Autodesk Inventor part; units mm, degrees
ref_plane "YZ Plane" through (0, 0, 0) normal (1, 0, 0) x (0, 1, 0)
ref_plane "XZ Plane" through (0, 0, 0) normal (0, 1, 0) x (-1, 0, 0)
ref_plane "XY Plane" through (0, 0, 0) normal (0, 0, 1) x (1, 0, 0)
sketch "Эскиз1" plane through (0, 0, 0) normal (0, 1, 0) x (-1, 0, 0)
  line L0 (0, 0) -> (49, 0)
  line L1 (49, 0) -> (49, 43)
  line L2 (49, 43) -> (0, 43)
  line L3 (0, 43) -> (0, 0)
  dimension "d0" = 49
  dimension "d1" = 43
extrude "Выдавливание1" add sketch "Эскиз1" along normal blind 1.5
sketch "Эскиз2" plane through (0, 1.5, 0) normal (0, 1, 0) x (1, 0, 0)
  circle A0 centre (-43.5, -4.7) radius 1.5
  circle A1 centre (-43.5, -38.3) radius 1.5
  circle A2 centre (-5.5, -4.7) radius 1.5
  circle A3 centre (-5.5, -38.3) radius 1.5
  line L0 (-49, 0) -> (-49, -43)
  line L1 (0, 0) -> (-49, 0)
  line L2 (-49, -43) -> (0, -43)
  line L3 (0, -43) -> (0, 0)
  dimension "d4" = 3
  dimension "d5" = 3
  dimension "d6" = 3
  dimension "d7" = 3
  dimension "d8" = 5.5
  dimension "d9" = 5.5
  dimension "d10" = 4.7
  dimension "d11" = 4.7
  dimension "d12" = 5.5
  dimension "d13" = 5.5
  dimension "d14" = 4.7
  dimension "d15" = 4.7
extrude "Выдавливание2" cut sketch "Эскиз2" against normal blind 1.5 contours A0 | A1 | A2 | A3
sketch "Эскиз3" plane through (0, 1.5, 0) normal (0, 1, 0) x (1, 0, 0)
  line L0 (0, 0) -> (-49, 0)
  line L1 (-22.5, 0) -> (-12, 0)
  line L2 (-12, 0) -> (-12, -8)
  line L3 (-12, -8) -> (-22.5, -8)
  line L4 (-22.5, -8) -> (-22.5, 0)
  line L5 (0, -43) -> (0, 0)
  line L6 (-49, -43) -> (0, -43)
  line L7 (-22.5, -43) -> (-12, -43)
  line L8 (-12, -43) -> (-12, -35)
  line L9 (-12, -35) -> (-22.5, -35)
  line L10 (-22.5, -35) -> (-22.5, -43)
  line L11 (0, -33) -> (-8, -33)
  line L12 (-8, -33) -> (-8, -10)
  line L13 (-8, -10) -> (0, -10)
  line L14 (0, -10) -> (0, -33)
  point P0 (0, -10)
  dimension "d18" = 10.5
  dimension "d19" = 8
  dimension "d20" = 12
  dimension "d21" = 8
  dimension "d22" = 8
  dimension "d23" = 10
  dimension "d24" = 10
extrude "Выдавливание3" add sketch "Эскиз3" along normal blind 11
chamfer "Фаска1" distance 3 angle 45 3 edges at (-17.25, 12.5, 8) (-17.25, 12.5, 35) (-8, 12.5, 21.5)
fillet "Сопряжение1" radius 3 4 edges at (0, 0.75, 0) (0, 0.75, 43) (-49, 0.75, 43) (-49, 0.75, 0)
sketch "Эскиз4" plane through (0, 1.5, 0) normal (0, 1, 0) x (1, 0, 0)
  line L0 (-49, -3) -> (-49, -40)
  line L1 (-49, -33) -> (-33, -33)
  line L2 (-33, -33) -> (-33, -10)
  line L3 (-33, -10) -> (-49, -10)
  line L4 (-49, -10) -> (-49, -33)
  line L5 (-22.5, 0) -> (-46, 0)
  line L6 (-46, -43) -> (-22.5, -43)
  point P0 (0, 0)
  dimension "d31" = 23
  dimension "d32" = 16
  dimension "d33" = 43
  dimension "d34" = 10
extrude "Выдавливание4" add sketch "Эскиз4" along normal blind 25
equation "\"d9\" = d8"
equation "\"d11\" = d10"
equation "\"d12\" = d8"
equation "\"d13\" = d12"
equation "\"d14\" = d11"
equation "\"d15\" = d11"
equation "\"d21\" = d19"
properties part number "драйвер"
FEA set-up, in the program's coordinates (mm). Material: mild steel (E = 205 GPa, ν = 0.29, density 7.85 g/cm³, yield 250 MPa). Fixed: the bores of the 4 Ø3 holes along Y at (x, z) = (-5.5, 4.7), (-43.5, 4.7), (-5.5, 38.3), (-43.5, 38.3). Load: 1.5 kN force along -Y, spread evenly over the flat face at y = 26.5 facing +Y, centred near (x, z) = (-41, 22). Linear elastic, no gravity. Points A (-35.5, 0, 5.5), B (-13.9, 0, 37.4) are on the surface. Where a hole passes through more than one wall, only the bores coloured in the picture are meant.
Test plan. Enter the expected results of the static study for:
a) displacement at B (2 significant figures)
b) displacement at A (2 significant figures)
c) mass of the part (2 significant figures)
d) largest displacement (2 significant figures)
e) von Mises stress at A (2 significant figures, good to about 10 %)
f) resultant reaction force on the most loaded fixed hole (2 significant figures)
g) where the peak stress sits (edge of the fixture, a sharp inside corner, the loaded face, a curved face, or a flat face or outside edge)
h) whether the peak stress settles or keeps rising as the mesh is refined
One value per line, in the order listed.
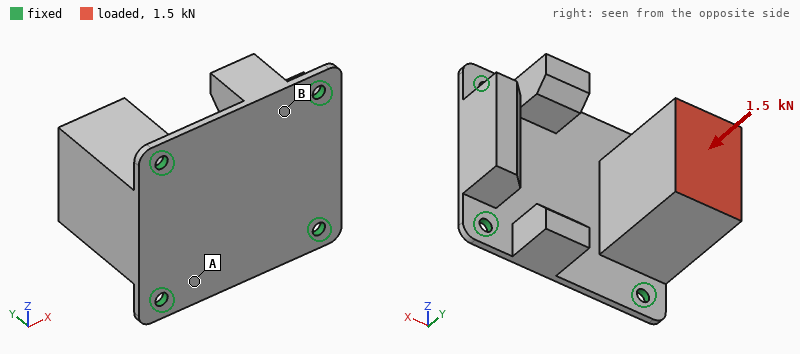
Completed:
9.2 µm
20 µm
130 g
54 µm
58 MPa
790 N
edge of the fixture
keeps rising
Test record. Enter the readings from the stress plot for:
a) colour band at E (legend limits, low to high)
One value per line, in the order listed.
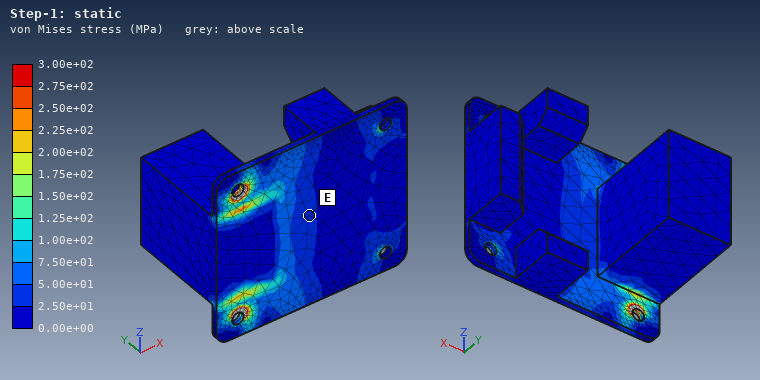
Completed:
2.50e+01 to 5.00e+01 MPa
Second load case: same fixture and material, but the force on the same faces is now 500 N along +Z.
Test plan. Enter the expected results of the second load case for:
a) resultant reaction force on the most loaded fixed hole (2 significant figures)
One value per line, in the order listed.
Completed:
510 N
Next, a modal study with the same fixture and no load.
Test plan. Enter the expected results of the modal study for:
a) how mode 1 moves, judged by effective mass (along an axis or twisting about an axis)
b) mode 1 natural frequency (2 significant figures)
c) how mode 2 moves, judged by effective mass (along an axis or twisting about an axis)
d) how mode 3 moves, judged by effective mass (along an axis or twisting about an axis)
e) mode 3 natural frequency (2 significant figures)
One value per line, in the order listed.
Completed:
along X
1400 Hz
along Z
along Y
4400 Hz
